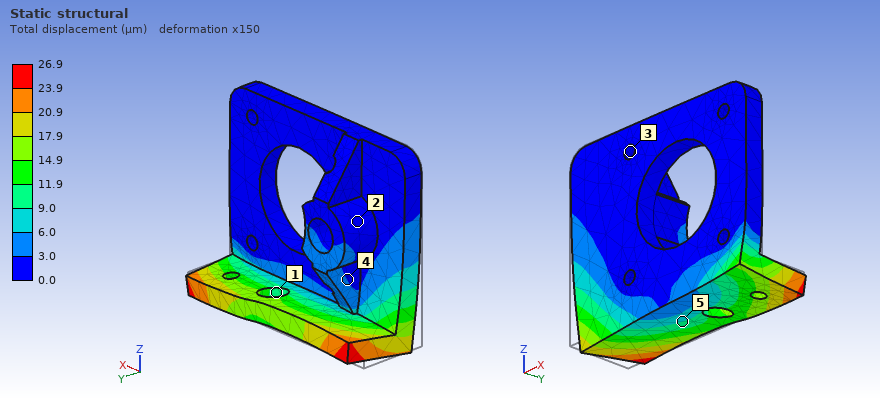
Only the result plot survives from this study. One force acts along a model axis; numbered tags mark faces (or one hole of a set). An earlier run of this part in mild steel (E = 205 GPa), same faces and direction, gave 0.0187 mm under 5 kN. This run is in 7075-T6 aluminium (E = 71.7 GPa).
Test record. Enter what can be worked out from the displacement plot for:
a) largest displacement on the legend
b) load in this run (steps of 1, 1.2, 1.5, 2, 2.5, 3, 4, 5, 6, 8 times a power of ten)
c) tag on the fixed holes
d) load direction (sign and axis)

26.9 µm
2.5 kN
3
+X
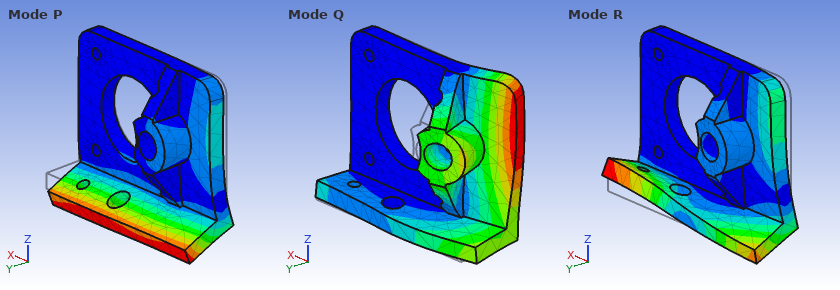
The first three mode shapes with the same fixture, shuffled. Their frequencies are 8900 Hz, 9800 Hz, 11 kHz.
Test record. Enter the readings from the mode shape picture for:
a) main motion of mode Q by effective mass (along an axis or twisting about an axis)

along Y
